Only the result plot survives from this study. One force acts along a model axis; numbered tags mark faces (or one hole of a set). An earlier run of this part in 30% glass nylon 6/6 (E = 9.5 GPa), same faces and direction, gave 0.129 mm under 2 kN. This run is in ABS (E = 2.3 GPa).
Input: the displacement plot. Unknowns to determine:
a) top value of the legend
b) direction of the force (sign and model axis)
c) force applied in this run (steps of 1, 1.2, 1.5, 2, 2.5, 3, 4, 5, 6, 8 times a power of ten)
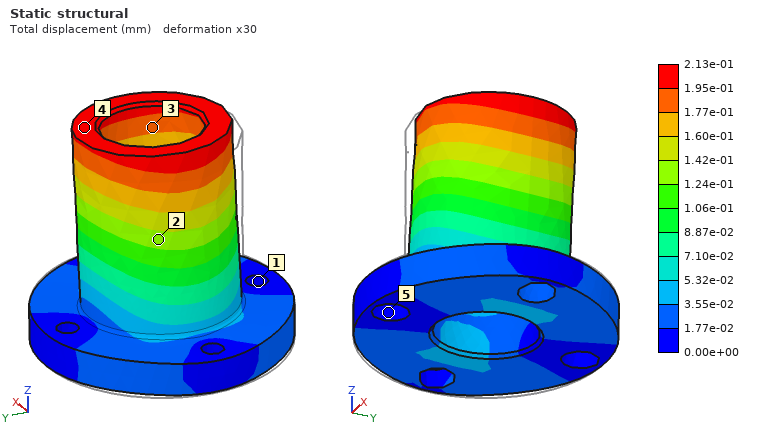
2.13e-01 mm
+X
800 N
